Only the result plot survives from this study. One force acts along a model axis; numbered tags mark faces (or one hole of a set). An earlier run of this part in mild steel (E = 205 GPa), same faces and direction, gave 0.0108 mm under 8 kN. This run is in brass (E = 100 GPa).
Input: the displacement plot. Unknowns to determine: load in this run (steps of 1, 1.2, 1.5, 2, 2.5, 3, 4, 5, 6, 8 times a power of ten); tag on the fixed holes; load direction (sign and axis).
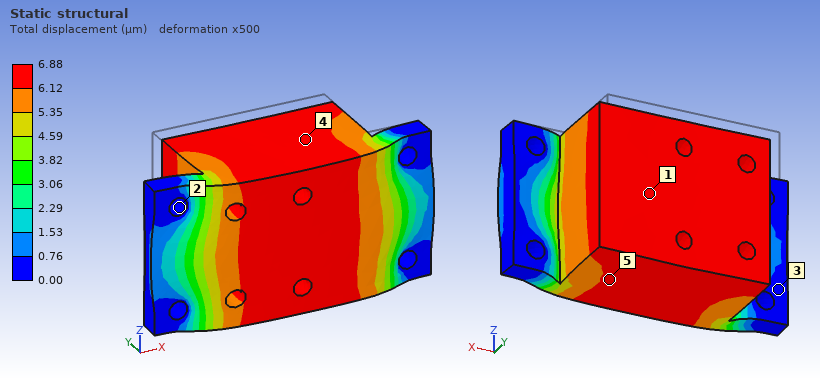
2.5 kN
2
-Y
